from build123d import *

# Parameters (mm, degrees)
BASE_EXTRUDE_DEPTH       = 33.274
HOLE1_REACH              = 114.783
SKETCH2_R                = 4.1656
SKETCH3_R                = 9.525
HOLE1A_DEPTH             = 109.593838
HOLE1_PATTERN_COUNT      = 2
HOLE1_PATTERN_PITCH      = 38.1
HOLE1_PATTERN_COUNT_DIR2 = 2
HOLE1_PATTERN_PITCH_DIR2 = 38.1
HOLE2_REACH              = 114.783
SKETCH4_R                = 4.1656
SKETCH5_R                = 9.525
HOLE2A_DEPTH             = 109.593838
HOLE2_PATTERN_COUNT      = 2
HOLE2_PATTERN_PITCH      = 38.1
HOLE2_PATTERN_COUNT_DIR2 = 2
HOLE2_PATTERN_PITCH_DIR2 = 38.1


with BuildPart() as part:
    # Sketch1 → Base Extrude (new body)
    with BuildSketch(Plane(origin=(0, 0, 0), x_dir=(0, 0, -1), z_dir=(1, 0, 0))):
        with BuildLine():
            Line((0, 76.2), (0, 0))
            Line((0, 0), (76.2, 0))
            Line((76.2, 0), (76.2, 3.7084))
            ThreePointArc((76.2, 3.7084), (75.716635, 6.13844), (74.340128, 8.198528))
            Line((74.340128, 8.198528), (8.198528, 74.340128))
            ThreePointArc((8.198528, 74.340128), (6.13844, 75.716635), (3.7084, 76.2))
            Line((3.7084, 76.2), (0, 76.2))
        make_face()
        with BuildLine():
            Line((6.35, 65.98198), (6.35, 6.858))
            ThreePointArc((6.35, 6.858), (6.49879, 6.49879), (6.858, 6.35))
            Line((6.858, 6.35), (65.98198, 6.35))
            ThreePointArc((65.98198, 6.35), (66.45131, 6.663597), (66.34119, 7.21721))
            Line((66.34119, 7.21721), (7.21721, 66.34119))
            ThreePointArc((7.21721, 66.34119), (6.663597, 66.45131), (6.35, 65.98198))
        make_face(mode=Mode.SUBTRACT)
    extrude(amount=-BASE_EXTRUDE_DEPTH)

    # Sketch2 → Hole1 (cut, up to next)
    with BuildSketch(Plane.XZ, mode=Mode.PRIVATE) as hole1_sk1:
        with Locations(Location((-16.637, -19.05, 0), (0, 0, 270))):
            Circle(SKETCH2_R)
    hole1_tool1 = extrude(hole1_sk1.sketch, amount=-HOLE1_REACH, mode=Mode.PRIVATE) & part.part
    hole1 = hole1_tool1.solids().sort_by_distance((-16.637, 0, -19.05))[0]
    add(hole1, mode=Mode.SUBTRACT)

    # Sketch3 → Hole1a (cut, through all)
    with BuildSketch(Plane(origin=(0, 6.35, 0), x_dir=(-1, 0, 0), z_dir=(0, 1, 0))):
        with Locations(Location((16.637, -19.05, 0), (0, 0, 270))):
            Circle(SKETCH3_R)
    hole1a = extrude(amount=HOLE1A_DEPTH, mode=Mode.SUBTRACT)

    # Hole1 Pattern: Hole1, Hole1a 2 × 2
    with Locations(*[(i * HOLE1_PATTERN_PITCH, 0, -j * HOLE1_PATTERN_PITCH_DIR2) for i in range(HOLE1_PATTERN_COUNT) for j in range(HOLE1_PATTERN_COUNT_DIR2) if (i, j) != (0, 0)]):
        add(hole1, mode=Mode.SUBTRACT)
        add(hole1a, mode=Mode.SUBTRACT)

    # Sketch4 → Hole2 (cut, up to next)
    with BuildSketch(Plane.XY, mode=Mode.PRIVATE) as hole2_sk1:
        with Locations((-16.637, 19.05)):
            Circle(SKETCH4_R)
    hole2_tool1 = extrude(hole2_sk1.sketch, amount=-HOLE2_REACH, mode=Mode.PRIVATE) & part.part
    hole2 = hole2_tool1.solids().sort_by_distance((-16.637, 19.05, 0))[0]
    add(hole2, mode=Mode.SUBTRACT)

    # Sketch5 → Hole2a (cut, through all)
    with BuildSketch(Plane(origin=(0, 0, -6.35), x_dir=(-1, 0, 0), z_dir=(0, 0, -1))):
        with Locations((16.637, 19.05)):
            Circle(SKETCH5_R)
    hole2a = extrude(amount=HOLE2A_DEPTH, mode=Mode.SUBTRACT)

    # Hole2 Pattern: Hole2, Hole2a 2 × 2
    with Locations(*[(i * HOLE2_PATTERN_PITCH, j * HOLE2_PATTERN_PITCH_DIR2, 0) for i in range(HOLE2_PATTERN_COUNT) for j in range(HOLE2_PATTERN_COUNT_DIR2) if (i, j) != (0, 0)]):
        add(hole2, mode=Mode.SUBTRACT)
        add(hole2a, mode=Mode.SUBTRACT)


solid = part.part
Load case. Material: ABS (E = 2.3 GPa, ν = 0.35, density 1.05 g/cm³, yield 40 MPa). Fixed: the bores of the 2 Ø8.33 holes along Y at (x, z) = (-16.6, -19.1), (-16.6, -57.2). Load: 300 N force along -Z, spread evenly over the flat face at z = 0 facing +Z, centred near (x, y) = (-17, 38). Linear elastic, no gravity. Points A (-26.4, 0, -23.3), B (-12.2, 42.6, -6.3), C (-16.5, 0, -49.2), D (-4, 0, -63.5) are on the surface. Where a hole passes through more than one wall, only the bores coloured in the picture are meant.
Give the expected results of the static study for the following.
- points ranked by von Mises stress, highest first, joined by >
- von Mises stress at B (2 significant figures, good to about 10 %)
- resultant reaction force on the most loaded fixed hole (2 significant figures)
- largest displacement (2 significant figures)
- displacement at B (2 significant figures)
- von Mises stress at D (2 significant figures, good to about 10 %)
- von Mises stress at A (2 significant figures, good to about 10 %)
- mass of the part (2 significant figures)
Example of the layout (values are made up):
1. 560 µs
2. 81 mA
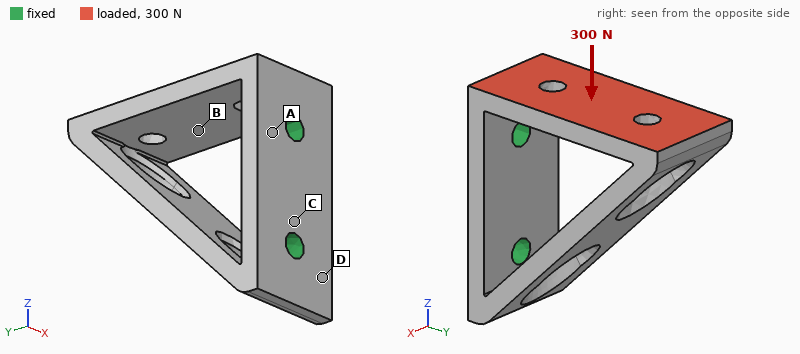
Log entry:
1. B > D > A > C
2. 6.5 MPa
3. 220 N
4. 0.73 mm
5. 0.69 mm
6. 4.2 MPa
7. 2.5 MPa
8. 45 g
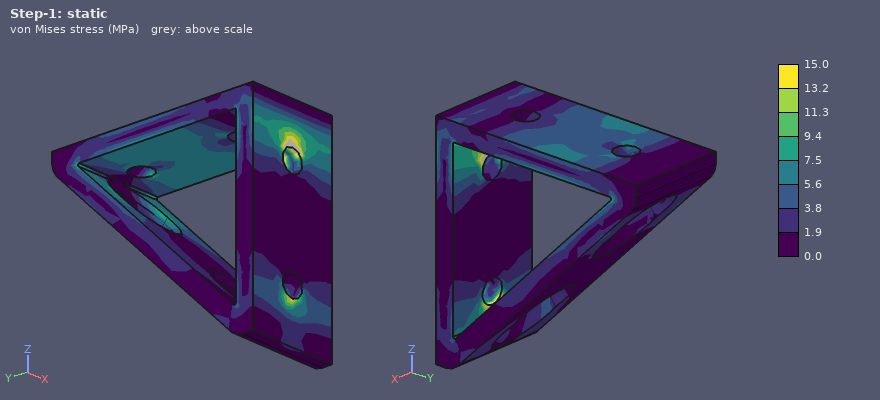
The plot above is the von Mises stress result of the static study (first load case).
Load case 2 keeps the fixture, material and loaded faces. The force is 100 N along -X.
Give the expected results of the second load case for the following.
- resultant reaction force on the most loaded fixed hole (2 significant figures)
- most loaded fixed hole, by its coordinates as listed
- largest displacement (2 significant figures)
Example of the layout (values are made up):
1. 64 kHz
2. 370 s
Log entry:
1. 120 N
2. (-16.6, -19.1)
3. 0.73 mm
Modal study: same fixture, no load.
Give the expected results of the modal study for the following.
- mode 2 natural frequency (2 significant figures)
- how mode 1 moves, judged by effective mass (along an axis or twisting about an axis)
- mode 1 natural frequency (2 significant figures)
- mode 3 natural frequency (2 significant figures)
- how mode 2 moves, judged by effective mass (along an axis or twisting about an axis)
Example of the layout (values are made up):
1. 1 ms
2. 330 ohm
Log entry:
1. 600 Hz
2. along X
3. 410 Hz
4. 1200 Hz
5. along Z
